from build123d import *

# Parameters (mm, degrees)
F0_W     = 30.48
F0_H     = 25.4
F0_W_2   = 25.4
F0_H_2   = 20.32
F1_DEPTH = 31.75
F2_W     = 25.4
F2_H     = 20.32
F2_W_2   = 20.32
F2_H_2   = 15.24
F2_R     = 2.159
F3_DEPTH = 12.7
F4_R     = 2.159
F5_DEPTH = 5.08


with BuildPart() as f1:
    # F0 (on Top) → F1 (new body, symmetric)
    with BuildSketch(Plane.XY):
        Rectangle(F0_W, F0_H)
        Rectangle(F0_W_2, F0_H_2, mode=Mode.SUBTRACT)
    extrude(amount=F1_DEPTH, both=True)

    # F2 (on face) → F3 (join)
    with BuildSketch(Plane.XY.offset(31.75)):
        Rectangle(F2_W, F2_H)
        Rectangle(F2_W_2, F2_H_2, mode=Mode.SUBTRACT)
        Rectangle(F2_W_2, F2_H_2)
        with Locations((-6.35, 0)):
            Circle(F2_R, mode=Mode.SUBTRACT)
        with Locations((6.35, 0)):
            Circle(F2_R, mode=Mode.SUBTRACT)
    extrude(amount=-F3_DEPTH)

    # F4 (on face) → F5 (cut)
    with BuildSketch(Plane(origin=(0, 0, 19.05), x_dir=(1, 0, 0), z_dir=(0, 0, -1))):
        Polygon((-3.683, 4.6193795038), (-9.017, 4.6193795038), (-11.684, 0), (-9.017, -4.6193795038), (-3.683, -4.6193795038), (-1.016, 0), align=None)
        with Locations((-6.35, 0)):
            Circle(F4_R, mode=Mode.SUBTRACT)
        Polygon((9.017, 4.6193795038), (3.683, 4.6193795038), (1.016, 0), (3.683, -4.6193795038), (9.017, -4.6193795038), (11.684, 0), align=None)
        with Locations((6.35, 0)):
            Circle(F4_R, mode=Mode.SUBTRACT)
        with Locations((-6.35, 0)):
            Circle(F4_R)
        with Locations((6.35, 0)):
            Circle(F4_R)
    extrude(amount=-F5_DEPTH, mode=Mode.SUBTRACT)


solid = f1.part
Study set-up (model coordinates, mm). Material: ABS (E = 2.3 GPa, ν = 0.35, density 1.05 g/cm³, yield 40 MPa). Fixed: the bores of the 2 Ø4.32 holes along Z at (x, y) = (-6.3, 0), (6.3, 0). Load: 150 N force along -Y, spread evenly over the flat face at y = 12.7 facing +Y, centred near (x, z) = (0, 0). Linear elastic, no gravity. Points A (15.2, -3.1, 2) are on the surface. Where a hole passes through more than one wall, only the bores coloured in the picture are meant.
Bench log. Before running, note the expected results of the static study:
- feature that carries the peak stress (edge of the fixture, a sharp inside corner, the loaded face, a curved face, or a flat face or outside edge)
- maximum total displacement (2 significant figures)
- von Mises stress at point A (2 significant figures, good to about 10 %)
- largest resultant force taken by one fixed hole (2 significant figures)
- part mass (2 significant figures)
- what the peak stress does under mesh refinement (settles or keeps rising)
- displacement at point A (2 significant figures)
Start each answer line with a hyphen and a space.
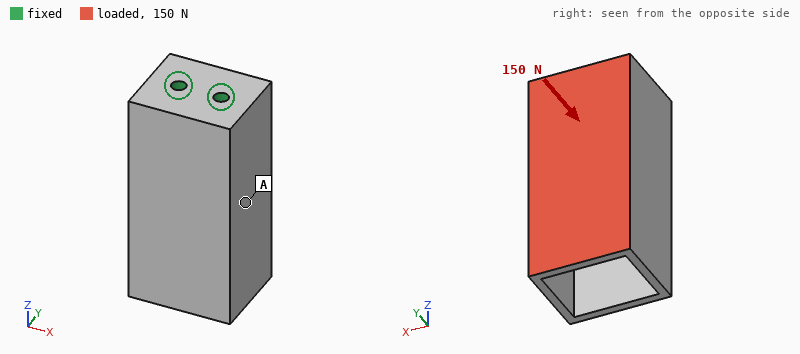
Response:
- edge of the fixture
- 0.45 mm
- 1.6 MPa
- 75 N
- 23 g
- keeps rising
- 0.15 mm
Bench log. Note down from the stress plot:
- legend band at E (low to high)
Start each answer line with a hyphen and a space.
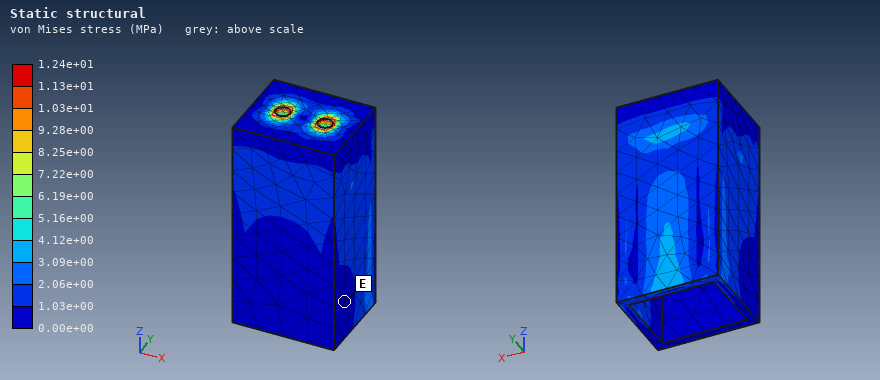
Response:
- 0.00e+00 to 1.03e+00 MPa
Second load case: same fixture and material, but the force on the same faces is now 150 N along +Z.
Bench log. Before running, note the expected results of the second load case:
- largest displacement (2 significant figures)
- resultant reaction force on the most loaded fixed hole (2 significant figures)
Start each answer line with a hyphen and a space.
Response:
- 0.17 mm
- 75 N
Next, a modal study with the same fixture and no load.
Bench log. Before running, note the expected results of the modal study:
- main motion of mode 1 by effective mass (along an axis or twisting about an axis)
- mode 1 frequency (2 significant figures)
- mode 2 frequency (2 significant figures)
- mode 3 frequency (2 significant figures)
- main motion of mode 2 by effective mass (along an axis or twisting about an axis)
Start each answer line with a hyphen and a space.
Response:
- along Y
- 930 Hz
- 1300 Hz
- 1900 Hz
- along X
